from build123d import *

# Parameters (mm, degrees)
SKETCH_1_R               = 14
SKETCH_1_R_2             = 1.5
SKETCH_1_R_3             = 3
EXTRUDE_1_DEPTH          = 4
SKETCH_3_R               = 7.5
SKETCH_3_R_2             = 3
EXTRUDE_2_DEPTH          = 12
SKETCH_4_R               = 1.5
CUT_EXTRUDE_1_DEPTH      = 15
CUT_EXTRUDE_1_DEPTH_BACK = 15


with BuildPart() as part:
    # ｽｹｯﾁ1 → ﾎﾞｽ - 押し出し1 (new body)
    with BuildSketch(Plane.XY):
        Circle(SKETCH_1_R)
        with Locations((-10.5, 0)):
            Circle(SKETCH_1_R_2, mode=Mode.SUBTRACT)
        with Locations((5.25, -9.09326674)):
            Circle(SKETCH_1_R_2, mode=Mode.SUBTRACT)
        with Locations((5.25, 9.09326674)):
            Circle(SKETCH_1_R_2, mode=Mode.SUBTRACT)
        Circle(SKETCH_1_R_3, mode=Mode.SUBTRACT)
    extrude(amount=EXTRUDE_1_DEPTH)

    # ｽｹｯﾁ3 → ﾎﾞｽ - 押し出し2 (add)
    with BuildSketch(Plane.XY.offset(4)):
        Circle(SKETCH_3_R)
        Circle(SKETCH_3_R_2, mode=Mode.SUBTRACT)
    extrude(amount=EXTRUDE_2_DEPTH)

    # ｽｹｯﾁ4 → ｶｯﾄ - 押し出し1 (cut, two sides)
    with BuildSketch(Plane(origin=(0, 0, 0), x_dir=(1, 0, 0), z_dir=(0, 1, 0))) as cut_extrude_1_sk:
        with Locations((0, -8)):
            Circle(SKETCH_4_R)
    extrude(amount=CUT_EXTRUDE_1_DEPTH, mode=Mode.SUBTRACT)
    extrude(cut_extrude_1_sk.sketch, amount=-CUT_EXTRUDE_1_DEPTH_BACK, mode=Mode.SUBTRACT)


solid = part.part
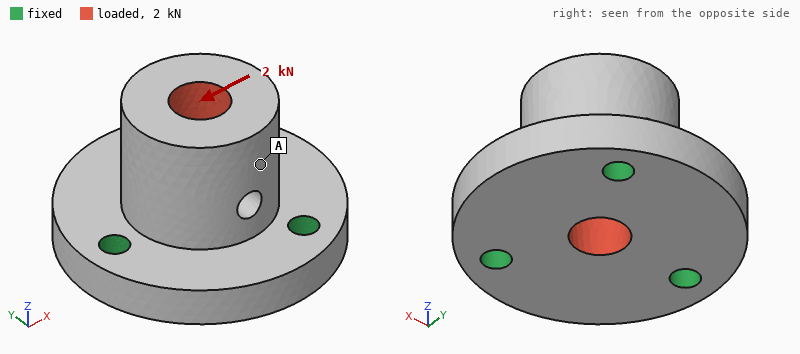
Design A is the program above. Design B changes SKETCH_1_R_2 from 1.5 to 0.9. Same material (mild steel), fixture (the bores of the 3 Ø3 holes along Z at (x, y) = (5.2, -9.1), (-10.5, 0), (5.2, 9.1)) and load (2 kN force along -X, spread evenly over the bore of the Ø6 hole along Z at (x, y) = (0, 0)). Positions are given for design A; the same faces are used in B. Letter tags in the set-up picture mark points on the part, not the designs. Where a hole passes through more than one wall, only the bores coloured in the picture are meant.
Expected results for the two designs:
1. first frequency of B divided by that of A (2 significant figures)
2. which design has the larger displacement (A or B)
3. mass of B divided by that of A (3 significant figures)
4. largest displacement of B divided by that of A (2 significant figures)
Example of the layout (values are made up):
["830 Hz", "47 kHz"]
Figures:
["0.90", "B", "1.01", "1.2"]
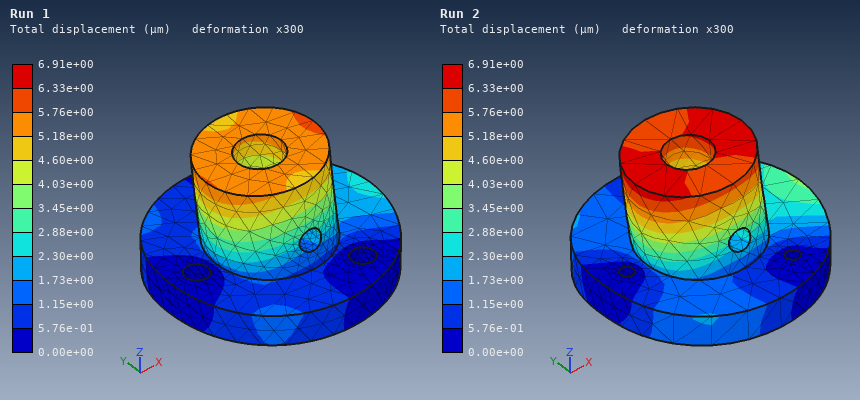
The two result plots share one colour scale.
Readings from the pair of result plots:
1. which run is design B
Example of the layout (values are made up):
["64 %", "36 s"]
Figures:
["Run 2"]
